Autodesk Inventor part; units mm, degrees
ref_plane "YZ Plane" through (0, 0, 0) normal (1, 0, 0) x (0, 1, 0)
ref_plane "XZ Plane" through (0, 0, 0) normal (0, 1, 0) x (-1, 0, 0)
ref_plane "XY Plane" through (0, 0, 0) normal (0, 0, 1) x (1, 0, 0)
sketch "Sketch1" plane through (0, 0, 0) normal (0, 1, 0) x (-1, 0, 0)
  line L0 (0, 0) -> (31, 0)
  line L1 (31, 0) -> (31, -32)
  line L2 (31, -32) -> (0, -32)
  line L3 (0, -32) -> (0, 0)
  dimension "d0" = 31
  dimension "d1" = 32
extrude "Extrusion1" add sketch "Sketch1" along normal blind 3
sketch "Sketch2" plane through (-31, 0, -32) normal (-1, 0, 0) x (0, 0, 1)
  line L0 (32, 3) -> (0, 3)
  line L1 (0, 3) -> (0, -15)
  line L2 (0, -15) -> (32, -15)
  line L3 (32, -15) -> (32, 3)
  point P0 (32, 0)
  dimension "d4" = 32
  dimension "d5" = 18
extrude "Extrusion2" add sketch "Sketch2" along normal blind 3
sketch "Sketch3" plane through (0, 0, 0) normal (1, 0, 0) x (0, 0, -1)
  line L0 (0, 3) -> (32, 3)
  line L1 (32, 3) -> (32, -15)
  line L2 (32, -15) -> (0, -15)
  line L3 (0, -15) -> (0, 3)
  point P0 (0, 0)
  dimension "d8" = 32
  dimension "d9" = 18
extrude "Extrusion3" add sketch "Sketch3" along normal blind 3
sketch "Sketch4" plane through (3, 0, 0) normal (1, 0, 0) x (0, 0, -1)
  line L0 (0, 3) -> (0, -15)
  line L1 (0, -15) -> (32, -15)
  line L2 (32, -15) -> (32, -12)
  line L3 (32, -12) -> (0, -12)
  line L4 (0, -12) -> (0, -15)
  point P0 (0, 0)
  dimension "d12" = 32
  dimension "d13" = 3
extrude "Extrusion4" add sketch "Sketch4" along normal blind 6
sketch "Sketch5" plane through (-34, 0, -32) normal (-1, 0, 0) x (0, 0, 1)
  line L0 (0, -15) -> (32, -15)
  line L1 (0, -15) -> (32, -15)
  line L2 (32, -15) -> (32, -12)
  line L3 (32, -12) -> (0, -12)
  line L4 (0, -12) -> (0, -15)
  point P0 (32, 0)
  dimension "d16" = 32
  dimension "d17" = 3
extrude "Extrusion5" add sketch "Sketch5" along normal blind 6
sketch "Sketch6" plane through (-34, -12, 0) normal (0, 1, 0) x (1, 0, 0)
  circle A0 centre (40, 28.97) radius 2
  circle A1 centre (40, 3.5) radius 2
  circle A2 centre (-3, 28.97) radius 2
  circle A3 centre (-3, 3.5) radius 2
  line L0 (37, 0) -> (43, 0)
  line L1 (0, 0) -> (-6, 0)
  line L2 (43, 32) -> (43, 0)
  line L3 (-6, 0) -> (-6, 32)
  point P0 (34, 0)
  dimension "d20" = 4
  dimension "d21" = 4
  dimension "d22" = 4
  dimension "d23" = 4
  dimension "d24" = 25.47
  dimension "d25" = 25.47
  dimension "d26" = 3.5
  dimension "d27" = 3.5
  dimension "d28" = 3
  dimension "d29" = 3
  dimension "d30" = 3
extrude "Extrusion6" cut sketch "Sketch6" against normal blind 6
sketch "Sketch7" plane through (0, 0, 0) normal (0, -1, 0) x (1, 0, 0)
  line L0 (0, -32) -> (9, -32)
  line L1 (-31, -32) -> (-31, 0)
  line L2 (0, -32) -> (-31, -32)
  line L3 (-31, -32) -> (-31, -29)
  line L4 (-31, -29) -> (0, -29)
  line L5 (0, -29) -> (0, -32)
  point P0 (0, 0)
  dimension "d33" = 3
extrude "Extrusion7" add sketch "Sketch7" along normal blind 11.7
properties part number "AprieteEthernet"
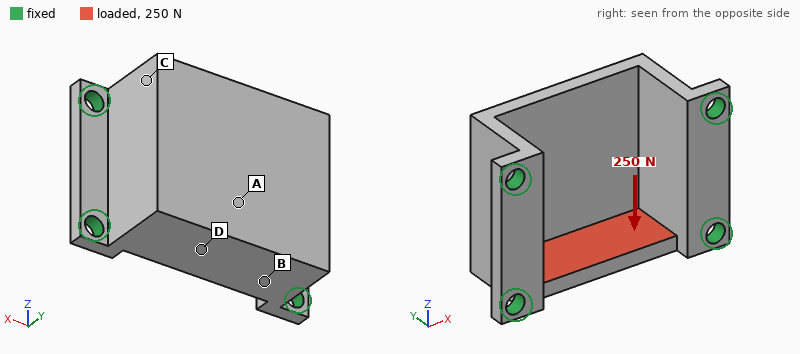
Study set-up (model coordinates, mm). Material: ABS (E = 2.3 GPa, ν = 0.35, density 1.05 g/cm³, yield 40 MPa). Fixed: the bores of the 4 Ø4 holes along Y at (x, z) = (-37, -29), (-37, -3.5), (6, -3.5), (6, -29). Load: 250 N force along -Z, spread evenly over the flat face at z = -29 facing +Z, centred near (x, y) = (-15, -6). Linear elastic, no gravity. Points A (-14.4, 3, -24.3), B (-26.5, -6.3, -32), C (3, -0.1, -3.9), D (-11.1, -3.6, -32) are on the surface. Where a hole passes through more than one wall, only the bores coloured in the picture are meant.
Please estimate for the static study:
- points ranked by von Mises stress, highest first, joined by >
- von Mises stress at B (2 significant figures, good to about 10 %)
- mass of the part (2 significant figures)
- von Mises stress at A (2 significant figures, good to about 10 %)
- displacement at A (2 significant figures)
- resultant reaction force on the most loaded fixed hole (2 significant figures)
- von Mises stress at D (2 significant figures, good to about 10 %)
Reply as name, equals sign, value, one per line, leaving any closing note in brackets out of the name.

points ranked by von Mises stress, highest first, joined by > = B > D > A > C
von Mises stress at B = 11 MPa
mass of the part = 8.9 g
von Mises stress at A = 4.0 MPa
displacement at A = 0.074 mm
resultant reaction force on the most loaded fixed hole = 77 N
von Mises stress at D = 7.4 MPa
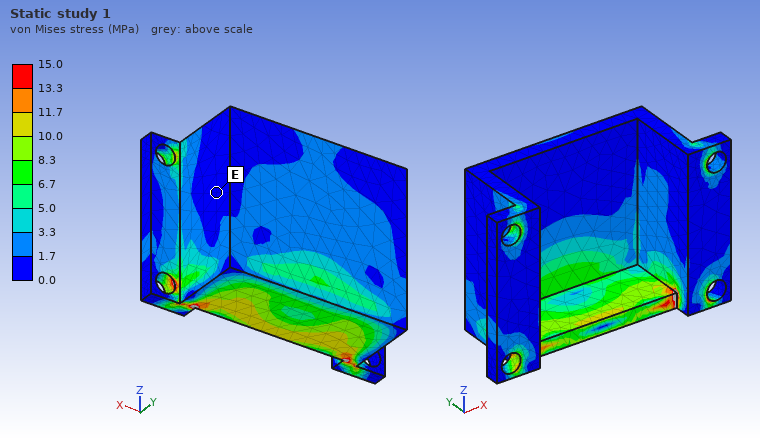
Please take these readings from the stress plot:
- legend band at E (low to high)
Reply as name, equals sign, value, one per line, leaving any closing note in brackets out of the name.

legend band at E = 0.0 to 1.7 MPa
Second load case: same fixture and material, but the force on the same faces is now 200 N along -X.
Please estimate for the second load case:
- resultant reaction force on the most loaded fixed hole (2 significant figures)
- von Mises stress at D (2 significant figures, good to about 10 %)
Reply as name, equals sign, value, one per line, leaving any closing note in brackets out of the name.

resultant reaction force on the most loaded fixed hole = 99 N
von Mises stress at D = 2.4 MPa
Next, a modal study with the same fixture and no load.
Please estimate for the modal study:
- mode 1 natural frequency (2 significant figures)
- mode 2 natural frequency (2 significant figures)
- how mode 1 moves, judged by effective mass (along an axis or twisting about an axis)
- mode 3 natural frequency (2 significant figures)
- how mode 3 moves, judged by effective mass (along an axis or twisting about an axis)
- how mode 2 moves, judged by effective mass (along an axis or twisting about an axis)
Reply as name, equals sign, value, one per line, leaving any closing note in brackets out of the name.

mode 1 natural frequency = 2800 Hz
mode 2 natural frequency = 3400 Hz
how mode 1 moves, judged by effective mass = along X
mode 3 natural frequency = 4000 Hz
how mode 3 moves, judged by effective mass = along Z
how mode 2 moves, judged by effective mass = along Y
